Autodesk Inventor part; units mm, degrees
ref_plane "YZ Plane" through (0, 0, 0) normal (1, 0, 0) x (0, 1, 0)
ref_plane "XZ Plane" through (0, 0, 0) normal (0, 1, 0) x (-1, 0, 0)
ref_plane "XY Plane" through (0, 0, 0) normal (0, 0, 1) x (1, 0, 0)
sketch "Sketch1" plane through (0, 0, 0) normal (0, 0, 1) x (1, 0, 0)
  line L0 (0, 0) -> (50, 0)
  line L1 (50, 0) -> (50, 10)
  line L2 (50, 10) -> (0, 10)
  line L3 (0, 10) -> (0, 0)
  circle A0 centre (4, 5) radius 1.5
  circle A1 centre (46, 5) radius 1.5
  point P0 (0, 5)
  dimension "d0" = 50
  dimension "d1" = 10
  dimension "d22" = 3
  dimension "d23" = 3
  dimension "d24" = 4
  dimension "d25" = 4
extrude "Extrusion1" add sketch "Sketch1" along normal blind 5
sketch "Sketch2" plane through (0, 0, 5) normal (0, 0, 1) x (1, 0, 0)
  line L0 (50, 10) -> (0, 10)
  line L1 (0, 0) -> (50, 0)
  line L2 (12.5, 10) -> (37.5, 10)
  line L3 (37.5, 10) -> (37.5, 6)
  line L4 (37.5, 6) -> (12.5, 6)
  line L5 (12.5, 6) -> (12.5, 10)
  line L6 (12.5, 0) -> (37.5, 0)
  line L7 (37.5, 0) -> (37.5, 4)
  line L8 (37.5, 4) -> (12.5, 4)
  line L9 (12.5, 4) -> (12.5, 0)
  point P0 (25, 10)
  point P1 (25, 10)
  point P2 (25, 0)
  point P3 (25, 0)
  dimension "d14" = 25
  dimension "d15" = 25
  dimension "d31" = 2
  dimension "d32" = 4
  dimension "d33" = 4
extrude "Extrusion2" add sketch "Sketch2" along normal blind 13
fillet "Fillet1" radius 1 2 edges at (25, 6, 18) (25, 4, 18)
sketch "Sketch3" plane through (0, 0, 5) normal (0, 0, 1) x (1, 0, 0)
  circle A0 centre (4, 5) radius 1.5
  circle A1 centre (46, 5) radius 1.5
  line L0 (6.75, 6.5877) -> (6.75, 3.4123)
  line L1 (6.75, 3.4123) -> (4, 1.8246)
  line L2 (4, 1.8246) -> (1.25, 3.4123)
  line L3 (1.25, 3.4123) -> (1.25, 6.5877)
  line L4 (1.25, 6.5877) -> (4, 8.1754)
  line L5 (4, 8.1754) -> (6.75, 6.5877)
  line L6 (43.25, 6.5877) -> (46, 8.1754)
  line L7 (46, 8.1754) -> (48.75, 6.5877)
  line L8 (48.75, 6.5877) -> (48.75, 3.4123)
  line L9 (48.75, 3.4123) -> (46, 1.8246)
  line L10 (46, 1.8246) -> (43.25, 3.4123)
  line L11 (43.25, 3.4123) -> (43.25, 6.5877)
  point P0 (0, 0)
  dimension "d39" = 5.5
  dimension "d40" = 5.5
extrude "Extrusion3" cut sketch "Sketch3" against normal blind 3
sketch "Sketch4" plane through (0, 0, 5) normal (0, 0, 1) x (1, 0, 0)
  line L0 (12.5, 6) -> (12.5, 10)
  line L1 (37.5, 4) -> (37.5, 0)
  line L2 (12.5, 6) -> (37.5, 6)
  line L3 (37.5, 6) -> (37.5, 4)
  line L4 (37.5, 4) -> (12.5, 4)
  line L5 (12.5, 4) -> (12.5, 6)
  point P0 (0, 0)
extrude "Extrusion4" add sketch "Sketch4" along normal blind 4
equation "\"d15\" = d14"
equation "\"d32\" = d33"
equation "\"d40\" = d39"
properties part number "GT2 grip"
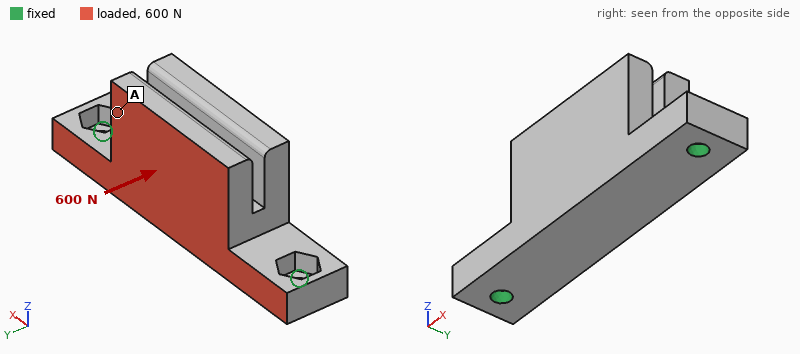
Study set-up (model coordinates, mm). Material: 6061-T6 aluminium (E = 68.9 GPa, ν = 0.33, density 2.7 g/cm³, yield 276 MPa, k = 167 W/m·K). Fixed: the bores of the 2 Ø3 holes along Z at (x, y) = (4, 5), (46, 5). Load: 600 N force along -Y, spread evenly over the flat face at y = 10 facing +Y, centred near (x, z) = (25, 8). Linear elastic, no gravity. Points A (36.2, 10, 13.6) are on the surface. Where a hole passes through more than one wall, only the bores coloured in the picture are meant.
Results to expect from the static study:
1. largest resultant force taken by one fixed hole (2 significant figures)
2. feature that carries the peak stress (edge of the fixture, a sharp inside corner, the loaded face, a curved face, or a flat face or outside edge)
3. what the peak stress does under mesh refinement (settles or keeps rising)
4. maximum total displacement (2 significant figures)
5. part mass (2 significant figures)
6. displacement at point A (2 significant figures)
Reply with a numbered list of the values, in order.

1. 300 N
2. edge of the fixture
3. keeps rising
4. 95 µm
5. 14 g
6. 71 µm
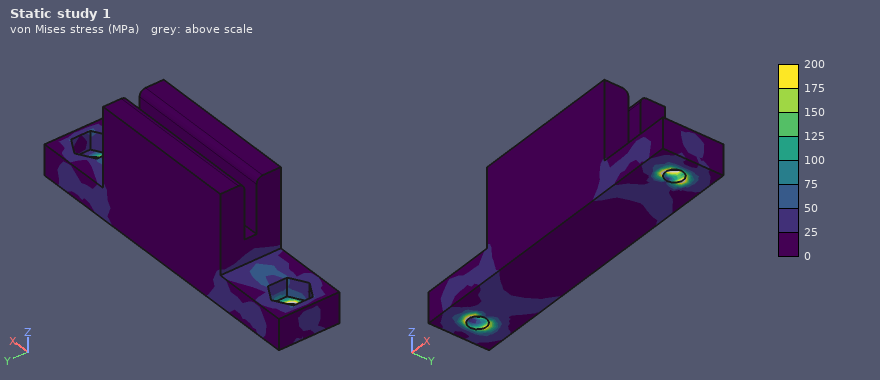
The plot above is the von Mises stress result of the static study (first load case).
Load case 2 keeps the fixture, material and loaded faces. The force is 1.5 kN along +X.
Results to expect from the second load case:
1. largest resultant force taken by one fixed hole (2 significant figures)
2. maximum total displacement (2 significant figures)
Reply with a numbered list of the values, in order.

1. 810 N
2. 14 µm
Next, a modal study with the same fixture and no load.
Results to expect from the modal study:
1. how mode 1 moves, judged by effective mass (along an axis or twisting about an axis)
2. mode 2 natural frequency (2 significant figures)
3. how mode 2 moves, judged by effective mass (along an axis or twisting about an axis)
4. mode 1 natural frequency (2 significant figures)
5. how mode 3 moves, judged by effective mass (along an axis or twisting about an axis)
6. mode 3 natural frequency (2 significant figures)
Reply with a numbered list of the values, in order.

1. along Y
2. 11 kHz
3. along Z
4. 4400 Hz
5. along Y
6. 17 kHz
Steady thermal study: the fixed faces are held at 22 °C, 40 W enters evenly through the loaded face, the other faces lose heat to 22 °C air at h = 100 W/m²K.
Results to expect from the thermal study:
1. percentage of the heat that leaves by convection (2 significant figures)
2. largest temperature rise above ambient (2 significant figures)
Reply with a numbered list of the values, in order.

1. 13 %
2. 35 K
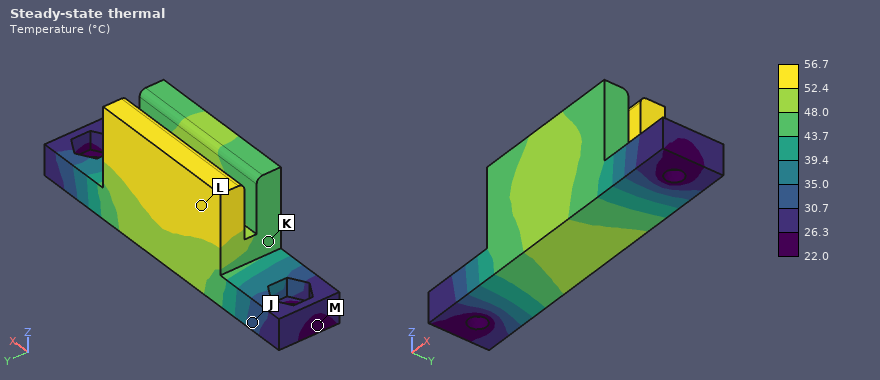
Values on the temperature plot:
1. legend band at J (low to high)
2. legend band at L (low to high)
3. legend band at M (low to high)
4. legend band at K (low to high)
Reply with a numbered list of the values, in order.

1. 30.7 to 35.0 °C
2. 52.4 to 56.7 °C
3. 22.0 to 26.3 °C
4. 43.7 to 48.0 °C
